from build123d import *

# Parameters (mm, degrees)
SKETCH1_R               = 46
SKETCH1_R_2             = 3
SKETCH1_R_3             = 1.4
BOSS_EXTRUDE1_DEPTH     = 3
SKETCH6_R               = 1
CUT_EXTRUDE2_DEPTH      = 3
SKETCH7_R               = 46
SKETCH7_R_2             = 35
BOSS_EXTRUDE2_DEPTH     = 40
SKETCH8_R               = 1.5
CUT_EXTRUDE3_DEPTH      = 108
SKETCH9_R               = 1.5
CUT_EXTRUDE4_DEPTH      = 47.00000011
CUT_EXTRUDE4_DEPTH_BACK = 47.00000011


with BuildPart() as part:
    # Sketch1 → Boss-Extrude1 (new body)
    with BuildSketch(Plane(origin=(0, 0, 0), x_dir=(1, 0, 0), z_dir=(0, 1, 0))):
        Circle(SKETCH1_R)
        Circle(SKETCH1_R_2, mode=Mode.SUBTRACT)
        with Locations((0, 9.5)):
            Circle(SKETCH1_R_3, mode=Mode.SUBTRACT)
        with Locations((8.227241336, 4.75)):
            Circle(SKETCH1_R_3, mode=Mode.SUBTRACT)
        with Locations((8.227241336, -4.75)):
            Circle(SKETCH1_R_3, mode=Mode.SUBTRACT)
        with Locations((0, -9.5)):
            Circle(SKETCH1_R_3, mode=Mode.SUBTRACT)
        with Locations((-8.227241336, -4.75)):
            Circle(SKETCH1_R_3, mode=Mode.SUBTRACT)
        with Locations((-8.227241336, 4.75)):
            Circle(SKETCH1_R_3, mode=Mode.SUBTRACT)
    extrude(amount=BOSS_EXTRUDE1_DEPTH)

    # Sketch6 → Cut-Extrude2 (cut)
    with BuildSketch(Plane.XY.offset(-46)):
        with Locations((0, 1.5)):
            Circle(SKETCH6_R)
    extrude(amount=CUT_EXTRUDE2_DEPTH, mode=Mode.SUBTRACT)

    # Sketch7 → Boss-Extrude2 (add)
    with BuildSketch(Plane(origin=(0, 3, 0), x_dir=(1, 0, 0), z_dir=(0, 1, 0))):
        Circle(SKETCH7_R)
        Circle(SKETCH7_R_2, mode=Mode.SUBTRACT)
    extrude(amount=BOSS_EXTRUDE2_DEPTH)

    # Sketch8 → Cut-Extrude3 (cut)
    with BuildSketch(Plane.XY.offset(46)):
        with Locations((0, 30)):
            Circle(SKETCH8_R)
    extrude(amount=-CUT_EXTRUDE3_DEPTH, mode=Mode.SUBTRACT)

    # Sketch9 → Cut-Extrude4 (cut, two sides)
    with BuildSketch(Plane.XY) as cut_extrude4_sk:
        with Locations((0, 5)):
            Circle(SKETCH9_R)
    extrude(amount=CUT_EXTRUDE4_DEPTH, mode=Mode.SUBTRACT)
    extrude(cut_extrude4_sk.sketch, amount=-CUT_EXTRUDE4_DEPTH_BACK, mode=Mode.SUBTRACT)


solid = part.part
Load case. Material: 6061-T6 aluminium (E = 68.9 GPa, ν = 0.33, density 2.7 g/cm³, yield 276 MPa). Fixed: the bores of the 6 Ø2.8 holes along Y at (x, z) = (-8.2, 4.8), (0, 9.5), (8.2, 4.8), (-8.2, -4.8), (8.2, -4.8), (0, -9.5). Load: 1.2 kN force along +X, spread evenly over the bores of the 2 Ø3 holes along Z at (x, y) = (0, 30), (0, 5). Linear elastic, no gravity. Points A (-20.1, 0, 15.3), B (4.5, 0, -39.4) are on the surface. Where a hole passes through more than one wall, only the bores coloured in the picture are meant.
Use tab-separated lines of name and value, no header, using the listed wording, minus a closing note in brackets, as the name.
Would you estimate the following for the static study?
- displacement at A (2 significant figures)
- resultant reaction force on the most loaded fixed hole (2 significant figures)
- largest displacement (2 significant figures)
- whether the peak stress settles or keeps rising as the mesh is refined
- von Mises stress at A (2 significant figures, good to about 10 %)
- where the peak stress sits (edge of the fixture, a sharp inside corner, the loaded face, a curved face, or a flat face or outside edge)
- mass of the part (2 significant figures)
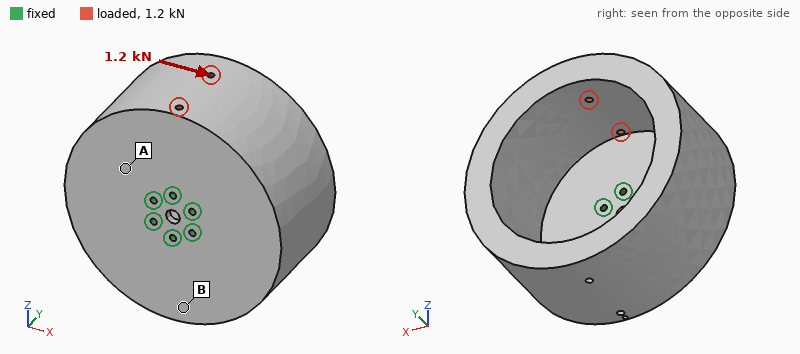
displacement at A	0.071 mm
resultant reaction force on the most loaded fixed hole	1.1 kN
largest displacement	0.27 mm
whether the peak stress settles or keeps rising as the mesh is refined	keeps rising
von Mises stress at A	18 MPa
where the peak stress sits	edge of the fixture
mass of the part	350 g
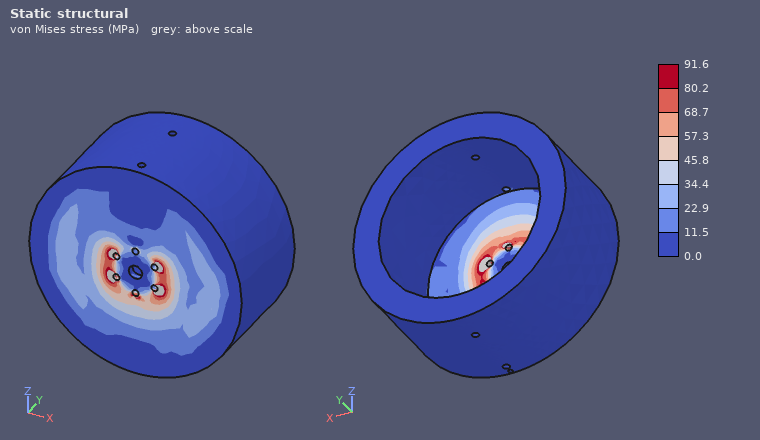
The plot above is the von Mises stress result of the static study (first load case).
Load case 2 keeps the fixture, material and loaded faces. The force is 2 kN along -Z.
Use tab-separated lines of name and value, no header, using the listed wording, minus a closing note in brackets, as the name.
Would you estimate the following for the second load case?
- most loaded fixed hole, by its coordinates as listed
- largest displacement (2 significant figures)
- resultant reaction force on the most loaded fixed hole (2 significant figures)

most loaded fixed hole, by its coordinates as listed	(0, 9.5)
largest displacement	0.47 mm
resultant reaction force on the most loaded fixed hole	740 N
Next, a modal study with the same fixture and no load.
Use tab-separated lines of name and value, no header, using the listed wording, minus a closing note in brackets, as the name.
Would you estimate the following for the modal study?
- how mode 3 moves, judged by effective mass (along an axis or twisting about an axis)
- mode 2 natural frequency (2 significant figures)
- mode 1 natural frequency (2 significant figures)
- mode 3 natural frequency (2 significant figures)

how mode 3 moves, judged by effective mass	along Y
mode 2 natural frequency	500 Hz
mode 1 natural frequency	490 Hz
mode 3 natural frequency	1100 Hz
